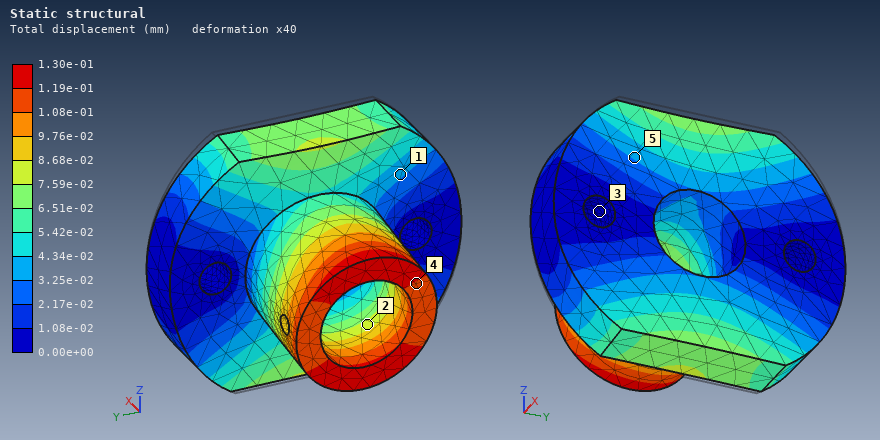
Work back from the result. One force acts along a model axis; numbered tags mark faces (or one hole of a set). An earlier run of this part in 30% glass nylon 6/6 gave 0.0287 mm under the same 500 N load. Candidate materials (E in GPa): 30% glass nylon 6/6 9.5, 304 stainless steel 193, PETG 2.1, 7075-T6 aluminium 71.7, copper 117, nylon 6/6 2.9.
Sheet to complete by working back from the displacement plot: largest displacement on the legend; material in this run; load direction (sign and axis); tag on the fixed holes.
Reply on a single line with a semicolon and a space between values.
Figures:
1.30e-01 mm; PETG; -Z; 3
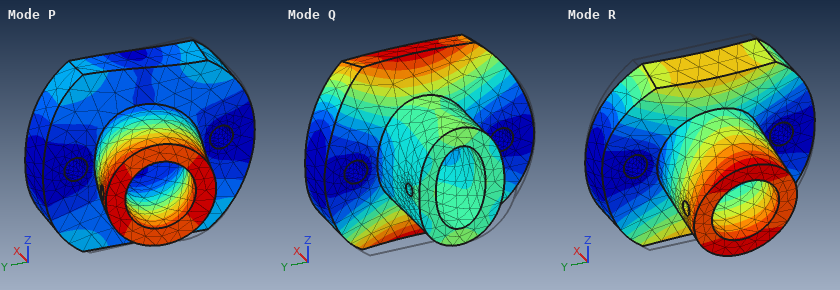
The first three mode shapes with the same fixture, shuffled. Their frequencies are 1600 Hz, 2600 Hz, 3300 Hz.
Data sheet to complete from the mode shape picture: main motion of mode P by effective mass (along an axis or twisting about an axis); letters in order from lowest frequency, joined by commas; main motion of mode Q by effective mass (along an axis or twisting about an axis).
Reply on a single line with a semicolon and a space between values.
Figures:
along Y; R, Q, P; along X
